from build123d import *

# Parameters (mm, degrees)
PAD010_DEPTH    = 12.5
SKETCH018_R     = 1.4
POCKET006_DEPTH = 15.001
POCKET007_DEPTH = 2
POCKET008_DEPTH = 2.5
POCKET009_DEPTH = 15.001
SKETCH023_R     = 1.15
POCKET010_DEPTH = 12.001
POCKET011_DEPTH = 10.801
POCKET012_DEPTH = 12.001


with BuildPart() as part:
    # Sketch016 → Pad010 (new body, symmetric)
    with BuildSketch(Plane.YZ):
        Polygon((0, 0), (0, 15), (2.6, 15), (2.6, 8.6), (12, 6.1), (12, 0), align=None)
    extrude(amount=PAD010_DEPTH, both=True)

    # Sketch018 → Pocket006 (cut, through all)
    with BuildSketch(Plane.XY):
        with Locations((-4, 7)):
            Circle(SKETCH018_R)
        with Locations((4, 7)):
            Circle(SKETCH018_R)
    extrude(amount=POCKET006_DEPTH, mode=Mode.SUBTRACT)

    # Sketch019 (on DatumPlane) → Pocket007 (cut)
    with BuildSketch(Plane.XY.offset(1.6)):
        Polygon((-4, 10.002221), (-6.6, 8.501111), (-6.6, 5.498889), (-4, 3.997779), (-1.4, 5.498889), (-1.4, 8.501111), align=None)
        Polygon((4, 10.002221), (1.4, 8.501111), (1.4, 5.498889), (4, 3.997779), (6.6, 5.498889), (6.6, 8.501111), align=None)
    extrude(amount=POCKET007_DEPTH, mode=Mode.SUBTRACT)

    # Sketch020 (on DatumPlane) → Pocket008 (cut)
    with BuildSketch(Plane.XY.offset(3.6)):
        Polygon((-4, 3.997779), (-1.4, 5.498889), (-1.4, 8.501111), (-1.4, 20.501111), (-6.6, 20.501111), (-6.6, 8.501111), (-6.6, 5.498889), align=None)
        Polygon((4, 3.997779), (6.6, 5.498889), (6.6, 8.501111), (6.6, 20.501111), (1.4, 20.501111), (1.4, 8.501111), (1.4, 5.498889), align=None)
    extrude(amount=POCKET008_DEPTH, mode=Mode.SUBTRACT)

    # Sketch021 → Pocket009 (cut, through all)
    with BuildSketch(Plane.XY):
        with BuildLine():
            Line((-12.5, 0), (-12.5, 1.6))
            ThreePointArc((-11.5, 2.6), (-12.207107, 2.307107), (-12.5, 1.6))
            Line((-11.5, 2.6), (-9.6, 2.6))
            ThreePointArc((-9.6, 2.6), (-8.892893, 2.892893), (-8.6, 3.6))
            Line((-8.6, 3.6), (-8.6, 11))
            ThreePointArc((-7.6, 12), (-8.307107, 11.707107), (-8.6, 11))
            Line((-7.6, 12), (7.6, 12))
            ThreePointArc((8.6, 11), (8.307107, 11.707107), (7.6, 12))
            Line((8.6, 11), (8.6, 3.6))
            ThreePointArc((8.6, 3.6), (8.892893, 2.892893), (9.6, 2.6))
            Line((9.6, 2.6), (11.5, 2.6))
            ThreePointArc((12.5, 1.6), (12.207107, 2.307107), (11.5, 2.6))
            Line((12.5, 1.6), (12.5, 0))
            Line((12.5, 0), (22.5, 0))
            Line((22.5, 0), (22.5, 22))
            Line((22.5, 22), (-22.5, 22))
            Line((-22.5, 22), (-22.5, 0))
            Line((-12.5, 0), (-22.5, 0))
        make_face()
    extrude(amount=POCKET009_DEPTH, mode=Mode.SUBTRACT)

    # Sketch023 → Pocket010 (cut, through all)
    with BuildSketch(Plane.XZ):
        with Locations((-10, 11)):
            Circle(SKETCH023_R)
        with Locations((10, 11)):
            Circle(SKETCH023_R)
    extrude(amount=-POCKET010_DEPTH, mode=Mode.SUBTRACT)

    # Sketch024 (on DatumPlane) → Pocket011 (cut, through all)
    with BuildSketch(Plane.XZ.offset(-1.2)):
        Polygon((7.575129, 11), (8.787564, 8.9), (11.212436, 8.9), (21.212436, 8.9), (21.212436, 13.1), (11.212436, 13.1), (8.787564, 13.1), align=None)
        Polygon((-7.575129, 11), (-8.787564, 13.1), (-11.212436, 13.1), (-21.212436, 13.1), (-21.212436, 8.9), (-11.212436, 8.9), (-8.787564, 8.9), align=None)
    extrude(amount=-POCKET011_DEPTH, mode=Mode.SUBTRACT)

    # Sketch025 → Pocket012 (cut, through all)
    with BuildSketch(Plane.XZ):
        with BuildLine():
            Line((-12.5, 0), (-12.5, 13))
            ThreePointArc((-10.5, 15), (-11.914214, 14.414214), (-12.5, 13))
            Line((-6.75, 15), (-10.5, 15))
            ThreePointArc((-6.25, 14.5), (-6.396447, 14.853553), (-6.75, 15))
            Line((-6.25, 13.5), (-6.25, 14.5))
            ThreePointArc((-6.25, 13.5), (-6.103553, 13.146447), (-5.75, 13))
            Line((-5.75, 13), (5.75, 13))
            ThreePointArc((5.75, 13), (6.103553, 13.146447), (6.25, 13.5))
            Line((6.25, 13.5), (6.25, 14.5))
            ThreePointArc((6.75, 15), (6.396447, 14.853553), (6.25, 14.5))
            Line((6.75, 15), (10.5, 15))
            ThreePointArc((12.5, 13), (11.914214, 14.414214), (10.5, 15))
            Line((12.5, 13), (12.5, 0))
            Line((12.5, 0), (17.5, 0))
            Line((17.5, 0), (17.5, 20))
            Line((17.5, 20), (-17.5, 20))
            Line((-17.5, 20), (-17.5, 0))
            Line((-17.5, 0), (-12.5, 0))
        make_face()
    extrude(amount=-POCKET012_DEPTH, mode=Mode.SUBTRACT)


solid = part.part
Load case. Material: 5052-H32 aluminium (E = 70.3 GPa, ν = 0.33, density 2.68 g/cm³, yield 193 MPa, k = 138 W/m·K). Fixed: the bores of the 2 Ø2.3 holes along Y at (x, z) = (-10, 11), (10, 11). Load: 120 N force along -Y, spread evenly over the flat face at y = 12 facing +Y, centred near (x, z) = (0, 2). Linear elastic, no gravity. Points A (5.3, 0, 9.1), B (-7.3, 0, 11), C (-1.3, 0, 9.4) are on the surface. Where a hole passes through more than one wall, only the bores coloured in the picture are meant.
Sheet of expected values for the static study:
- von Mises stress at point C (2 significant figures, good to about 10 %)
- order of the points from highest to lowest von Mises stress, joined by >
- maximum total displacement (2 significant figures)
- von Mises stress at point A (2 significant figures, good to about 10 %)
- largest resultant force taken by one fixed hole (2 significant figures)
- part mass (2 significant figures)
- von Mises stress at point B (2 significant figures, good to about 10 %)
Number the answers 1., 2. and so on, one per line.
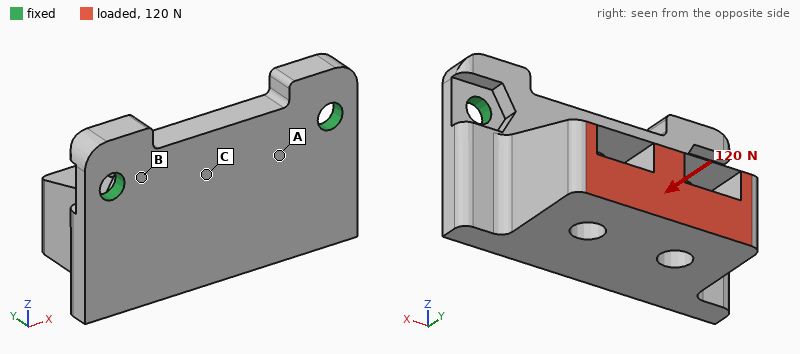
1. 13 MPa
2. B > A > C
3. 78 µm
4. 32 MPa
5. 60 N
6. 4.6 g
7. 52 MPa
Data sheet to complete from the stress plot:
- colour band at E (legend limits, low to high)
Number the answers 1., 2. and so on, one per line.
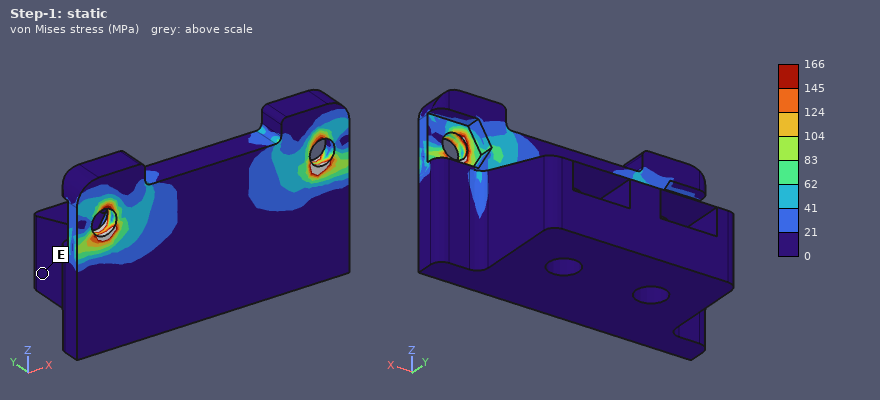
1. 0 to 21 MPa
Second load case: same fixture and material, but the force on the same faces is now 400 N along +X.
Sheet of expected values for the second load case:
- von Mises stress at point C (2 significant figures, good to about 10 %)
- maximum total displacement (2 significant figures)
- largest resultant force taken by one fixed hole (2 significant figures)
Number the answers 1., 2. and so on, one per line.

1. 11 MPa
2. 22 µm
3. 350 N
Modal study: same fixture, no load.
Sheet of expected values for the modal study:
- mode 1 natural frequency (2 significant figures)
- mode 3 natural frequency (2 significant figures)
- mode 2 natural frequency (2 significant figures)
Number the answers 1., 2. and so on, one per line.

1. 4000 Hz
2. 25 kHz
3. 19 kHz
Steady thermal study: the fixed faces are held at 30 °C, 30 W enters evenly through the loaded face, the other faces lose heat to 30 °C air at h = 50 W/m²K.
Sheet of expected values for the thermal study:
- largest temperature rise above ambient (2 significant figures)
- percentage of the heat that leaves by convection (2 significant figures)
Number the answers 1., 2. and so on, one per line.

1. 66 K
2. 9.2 %
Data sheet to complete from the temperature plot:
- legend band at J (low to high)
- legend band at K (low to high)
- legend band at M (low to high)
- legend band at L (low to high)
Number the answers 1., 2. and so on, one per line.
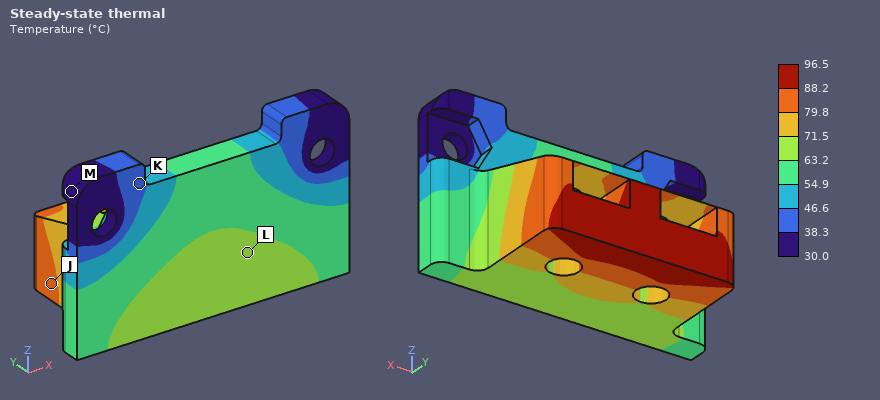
1. 79.8 to 88.2 °C
2. 38.3 to 46.6 °C
3. 30.0 to 38.3 °C
4. 63.2 to 71.5 °C
